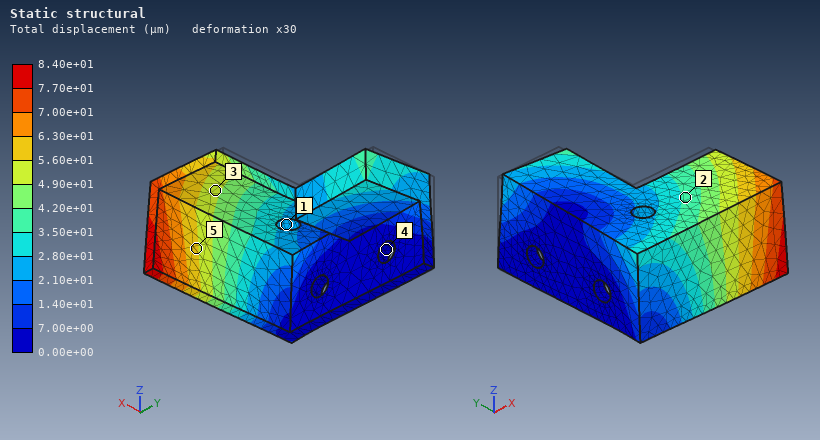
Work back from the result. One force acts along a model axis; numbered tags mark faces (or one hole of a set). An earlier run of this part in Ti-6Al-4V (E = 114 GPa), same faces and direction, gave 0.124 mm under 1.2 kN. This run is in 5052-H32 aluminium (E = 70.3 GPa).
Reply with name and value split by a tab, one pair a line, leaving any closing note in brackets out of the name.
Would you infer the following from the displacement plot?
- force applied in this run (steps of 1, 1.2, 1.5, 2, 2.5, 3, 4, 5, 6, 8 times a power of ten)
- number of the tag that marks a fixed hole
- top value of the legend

force applied in this run	500 N
number of the tag that marks a fixed hole	4
top value of the legend	8.40e+01 µm
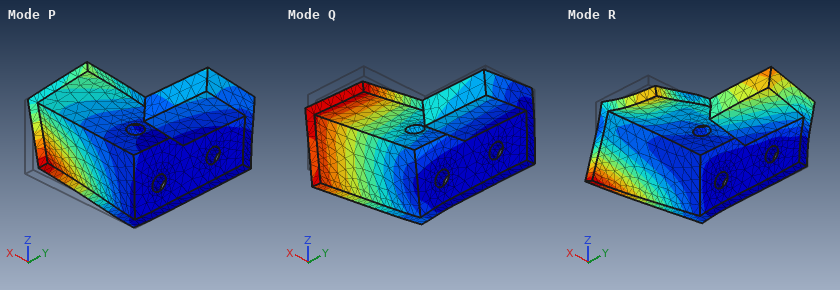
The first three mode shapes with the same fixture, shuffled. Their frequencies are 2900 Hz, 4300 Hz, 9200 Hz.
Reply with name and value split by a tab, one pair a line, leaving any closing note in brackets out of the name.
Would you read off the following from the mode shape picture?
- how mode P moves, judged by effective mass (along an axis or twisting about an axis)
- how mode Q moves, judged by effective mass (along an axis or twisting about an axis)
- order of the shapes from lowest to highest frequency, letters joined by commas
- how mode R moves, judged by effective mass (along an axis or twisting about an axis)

how mode P moves, judged by effective mass	along Y
how mode Q moves, judged by effective mass	along Z
order of the shapes from lowest to highest frequency, letters joined by commas	Q, P, R
how mode R moves, judged by effective mass	along X
